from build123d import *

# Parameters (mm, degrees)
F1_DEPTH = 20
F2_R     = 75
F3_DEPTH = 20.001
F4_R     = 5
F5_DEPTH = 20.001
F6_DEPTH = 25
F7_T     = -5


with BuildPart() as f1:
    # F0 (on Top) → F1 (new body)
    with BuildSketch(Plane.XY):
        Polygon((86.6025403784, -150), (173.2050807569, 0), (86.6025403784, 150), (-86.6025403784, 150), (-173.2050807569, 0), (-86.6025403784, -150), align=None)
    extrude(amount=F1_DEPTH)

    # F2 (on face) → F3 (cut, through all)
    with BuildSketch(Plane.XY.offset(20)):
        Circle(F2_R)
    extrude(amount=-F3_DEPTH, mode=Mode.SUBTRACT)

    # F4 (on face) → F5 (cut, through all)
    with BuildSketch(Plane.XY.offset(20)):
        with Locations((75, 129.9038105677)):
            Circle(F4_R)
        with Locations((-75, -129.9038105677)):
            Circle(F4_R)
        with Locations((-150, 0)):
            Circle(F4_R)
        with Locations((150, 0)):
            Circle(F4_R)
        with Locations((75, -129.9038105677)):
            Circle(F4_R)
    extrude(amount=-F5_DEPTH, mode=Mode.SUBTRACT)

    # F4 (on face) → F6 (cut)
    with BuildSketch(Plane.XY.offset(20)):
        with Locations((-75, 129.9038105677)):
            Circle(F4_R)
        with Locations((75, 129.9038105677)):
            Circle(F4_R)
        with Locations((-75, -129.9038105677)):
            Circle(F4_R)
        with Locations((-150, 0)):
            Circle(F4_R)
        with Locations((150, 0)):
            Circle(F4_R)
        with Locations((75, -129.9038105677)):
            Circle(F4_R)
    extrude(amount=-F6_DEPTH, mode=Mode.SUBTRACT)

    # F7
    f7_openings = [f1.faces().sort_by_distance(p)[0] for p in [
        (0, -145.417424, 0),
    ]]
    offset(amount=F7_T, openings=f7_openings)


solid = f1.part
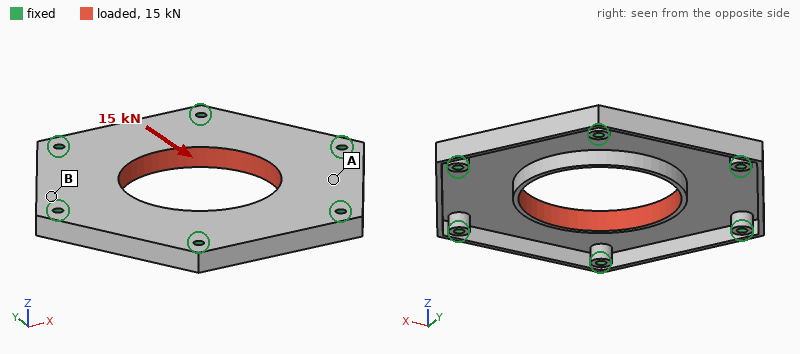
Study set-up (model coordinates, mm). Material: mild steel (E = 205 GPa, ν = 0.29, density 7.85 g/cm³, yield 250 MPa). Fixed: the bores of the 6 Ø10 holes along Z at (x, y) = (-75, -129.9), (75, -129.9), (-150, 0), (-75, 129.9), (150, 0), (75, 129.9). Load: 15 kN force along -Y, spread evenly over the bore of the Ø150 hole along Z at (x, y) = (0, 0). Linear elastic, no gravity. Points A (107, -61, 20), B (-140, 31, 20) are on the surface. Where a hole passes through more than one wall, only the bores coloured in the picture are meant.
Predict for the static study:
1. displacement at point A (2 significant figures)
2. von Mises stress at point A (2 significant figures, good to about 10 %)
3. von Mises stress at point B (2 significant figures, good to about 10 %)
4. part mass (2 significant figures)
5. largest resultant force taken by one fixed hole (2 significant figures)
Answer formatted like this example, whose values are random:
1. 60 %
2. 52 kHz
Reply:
1. 8.6 µm
2. 2.8 MPa
3. 5.5 MPa
4. 3.4 kg
5. 3.0 kN
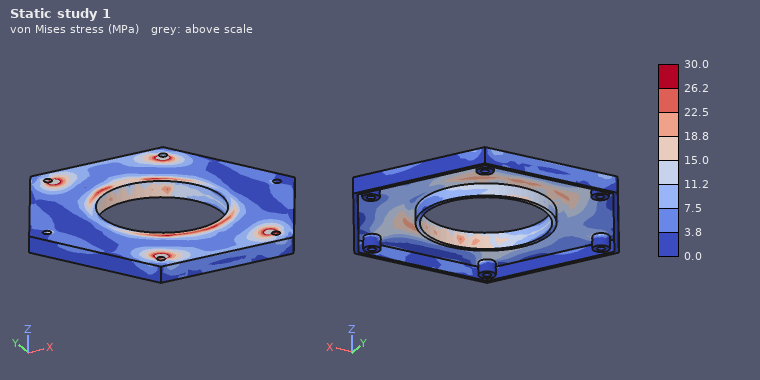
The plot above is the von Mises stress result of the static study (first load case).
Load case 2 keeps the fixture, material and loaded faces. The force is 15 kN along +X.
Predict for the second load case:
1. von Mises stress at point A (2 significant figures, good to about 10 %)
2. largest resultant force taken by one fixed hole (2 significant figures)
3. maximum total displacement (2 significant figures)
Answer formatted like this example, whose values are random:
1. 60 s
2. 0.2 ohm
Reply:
1. 4.6 MPa
2. 3.4 kN
3. 29 µm
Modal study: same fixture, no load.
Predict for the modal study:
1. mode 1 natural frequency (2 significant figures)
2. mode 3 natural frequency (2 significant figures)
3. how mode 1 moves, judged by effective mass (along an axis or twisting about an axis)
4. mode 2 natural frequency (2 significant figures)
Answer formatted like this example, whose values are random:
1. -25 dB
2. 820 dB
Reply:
1. 910 Hz
2. 1300 Hz
3. along Z
4. 1300 Hz
